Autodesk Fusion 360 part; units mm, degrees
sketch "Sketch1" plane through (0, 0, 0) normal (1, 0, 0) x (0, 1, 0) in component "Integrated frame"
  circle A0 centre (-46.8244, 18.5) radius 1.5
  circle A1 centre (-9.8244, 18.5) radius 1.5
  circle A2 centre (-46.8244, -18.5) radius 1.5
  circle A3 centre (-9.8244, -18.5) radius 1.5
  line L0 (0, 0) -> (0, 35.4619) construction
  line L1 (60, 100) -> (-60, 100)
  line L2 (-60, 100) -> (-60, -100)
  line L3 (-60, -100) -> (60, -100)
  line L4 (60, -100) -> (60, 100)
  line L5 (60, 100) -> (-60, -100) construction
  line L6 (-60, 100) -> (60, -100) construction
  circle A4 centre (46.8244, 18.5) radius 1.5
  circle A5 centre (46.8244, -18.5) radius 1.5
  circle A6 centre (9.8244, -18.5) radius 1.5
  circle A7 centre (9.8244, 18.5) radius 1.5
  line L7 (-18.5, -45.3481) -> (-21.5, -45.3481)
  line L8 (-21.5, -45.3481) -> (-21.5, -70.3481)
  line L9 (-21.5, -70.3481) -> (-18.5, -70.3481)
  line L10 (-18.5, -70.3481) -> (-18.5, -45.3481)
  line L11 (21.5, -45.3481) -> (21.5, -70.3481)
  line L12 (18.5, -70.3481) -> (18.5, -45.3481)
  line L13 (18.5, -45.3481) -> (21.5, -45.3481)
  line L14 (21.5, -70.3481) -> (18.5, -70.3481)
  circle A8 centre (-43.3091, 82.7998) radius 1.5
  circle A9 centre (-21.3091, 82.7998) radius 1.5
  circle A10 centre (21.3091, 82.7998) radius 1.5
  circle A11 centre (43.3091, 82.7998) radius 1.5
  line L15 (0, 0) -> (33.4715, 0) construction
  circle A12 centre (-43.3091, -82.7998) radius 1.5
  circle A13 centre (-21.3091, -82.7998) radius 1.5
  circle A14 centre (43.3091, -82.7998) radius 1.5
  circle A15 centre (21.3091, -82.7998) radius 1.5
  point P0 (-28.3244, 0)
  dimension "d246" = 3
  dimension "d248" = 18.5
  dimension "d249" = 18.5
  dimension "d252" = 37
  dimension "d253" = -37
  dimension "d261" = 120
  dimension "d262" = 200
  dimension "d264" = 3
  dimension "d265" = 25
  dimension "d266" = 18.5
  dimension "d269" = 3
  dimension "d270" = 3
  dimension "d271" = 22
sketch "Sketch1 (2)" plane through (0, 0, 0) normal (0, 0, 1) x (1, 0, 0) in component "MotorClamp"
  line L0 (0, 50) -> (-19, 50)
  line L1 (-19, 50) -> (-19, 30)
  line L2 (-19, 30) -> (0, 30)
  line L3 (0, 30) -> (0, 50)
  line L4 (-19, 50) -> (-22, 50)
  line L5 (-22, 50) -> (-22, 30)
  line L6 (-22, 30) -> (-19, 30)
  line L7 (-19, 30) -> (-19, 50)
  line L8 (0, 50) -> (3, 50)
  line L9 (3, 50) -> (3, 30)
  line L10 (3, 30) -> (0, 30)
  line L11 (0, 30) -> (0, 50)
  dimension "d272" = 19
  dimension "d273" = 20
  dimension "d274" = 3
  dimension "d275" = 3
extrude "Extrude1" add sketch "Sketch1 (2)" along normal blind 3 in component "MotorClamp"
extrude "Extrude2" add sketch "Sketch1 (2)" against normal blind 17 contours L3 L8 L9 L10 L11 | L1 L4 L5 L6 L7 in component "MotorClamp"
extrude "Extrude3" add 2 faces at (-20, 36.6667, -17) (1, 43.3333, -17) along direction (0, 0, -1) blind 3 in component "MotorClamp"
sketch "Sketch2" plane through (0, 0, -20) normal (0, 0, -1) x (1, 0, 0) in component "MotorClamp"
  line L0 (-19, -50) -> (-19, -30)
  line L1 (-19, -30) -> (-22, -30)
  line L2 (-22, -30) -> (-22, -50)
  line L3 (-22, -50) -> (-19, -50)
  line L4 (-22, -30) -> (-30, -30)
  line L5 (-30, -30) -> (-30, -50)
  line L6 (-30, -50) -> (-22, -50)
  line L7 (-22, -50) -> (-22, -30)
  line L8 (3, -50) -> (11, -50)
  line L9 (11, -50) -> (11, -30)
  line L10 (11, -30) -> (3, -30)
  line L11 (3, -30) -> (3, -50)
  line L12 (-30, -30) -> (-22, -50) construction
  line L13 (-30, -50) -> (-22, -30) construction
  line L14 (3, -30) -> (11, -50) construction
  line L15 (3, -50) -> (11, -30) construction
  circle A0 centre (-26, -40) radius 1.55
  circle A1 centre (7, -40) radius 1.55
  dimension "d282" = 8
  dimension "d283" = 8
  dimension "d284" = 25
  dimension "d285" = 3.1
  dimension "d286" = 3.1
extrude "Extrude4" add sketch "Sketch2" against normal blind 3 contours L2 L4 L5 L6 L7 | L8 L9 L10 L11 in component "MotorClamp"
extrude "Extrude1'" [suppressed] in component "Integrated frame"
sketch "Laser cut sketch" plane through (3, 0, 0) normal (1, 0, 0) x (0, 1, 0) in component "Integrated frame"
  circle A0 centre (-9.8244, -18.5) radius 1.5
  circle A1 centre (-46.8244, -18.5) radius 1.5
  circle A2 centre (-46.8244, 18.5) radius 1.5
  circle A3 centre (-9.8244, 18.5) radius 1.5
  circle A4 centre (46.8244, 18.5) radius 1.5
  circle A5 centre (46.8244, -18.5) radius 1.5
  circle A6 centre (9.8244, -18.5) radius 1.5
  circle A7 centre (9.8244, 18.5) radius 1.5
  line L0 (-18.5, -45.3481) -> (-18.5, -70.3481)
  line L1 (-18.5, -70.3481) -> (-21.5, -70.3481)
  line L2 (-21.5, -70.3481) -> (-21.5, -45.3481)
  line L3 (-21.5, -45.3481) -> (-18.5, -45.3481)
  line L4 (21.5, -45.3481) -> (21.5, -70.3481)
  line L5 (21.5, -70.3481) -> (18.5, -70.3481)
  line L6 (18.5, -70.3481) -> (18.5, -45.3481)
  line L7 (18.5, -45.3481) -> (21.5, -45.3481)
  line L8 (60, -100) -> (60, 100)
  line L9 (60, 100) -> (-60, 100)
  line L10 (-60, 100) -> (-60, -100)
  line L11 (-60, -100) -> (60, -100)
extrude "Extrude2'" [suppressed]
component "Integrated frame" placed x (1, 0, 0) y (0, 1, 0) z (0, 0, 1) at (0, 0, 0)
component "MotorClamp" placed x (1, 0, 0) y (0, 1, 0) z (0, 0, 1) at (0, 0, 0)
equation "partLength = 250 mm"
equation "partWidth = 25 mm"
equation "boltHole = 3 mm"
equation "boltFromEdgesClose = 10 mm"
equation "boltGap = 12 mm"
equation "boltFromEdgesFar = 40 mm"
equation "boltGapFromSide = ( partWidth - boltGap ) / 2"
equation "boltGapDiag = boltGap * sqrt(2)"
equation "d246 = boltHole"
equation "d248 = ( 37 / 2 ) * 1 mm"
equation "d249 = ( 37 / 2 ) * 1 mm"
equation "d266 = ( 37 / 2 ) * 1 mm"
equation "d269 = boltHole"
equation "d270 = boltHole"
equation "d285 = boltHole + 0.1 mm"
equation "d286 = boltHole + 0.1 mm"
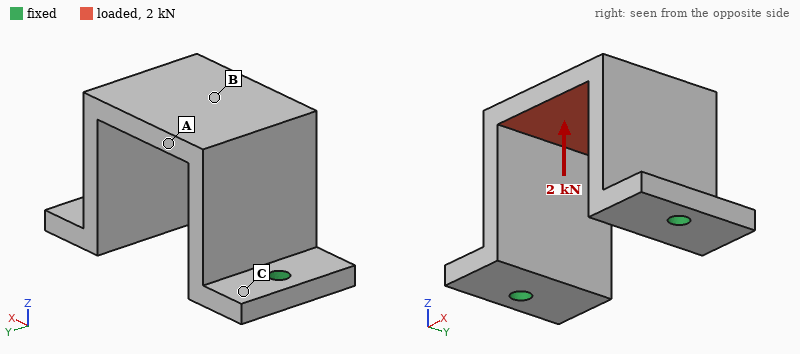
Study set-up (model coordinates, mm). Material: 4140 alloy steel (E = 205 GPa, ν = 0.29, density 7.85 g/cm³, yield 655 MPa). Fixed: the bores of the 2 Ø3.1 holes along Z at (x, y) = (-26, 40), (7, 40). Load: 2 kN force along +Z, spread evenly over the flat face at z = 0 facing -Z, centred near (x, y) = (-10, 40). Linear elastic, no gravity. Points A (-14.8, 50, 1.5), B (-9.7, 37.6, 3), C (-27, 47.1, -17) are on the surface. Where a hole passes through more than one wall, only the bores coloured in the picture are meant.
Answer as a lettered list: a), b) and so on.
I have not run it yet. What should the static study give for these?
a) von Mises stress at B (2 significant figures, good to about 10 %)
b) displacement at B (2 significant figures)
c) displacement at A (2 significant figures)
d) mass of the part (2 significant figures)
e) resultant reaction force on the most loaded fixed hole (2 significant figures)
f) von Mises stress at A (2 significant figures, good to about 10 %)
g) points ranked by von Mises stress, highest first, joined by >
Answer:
a) 94 MPa
b) 19 µm
c) 16 µm
d) 38 g
e) 1.0 kN
f) 43 MPa
g) B > A > C
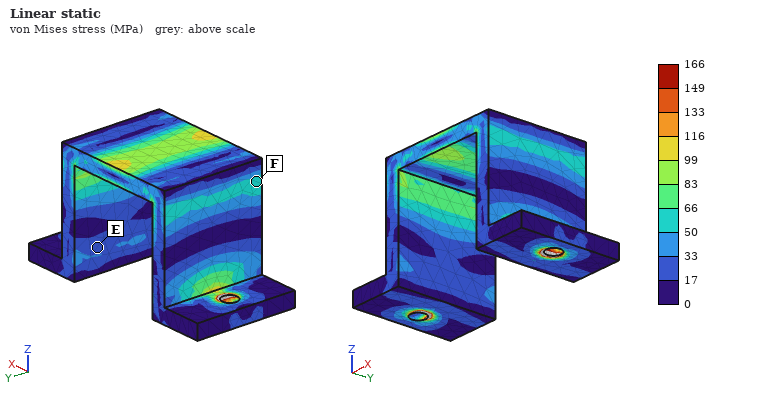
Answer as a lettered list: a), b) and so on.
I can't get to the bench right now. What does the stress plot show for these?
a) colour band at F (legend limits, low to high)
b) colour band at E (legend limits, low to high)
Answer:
a) 50 to 66 MPa
b) 17 to 33 MPa
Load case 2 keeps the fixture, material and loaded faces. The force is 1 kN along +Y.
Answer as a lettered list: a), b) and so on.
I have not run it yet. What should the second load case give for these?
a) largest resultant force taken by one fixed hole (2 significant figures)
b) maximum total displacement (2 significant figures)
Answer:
a) 500 N
b) 94 µm
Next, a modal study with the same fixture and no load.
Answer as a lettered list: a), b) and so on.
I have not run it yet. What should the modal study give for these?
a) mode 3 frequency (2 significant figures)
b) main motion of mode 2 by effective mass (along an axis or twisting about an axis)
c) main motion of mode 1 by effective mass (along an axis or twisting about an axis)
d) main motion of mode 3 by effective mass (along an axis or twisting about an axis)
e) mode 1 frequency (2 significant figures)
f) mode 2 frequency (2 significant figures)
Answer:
a) 7000 Hz
b) along X
c) along Y
d) twisting about Z
e) 3900 Hz
f) 4700 Hz
